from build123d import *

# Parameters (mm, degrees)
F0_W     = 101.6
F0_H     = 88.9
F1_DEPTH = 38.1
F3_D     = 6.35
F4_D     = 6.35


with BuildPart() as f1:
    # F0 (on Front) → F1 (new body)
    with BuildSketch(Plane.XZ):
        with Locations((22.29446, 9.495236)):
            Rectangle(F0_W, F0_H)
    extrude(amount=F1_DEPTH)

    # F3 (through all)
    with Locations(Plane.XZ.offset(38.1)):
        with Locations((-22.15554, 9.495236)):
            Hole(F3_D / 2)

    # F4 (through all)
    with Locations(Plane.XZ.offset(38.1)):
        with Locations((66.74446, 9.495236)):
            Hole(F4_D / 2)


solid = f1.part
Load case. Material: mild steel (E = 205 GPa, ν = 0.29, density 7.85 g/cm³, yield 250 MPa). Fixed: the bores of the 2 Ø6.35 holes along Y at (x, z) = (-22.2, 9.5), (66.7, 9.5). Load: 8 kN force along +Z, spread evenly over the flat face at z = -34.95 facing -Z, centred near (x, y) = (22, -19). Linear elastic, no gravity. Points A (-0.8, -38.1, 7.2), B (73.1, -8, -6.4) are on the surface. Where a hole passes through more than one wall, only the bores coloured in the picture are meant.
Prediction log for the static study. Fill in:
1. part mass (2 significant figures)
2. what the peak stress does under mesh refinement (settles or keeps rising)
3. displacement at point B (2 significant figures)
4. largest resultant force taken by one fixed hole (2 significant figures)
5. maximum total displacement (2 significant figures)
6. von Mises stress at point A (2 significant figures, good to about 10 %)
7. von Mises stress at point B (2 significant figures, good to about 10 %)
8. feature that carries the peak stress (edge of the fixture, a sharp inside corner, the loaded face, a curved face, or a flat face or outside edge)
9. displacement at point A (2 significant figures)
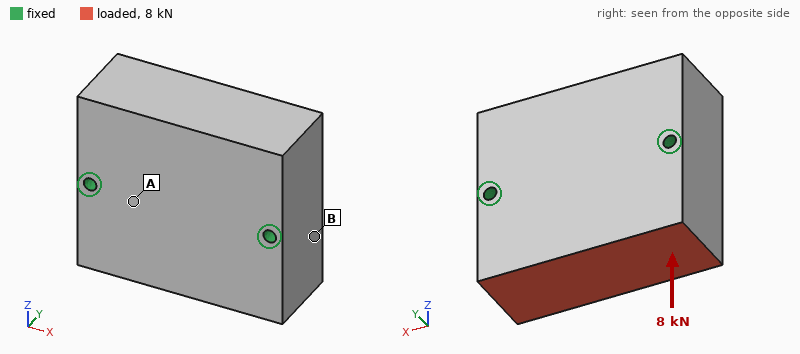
2.7 kg
keeps rising
0.26 µm
4.0 kN
0.90 µm
1.3 MPa
3.3 MPa
edge of the fixture
0.49 µm
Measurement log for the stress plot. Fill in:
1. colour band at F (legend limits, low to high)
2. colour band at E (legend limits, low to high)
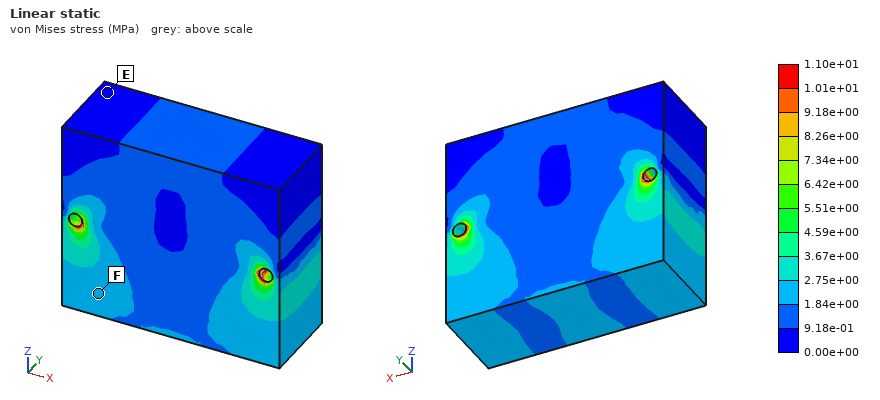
1.84e+00 to 2.75e+00 MPa
0.00e+00 to 9.18e-01 MPa
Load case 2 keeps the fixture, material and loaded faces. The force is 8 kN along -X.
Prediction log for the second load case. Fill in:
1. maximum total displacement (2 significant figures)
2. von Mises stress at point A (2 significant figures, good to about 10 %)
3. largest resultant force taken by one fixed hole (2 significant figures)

2.5 µm
2.9 MPa
5.6 kN
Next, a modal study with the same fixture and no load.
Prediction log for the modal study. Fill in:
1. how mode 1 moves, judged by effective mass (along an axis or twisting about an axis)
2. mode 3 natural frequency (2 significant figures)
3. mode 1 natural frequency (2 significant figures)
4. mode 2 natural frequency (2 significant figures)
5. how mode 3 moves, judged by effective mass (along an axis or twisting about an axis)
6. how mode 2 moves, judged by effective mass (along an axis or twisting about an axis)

twisting about X
12 kHz
6500 Hz
7900 Hz
along X
along Y
